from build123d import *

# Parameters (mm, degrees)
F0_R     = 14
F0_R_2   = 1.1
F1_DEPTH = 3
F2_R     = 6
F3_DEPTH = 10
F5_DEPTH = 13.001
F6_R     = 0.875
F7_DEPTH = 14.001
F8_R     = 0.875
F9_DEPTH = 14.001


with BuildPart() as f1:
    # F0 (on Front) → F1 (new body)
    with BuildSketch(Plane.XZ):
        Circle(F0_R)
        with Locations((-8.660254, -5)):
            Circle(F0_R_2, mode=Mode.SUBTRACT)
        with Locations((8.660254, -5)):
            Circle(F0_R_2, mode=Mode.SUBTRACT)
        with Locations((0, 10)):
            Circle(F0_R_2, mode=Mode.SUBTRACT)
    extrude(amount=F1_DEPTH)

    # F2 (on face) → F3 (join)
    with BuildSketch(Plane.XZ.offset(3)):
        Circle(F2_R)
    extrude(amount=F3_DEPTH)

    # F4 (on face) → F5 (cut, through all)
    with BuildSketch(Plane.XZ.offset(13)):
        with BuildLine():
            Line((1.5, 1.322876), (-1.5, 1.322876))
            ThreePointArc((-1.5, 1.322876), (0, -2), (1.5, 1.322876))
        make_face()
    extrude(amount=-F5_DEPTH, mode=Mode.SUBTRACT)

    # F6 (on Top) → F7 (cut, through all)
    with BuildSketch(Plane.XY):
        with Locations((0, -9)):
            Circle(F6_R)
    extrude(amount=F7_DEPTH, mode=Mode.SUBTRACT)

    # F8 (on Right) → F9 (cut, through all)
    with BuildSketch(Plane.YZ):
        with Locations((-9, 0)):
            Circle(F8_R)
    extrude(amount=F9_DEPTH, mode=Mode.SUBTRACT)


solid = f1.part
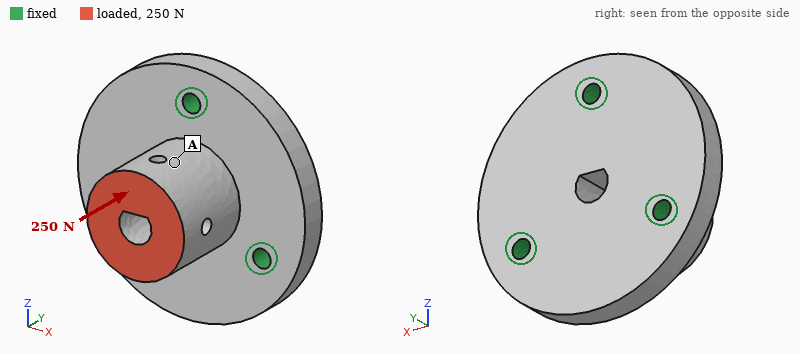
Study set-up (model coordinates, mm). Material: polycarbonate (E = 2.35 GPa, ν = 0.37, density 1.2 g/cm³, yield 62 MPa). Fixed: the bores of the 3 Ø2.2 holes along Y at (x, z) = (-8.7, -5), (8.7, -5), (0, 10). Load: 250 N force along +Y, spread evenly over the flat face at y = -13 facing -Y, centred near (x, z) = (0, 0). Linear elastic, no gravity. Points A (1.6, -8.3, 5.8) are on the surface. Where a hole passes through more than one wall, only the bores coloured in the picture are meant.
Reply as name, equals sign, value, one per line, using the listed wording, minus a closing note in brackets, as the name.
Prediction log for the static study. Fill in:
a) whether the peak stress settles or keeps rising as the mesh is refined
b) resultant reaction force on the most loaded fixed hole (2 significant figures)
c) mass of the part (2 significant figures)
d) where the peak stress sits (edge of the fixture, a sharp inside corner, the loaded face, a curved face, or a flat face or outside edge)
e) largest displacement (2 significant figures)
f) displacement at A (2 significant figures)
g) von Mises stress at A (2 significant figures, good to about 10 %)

whether the peak stress settles or keeps rising as the mesh is refined = keeps rising
resultant reaction force on the most loaded fixed hole = 86 N
mass of the part = 3.3 g
where the peak stress sits = edge of the fixture
largest displacement = 54 µm
displacement at A = 48 µm
von Mises stress at A = 3.4 MPa
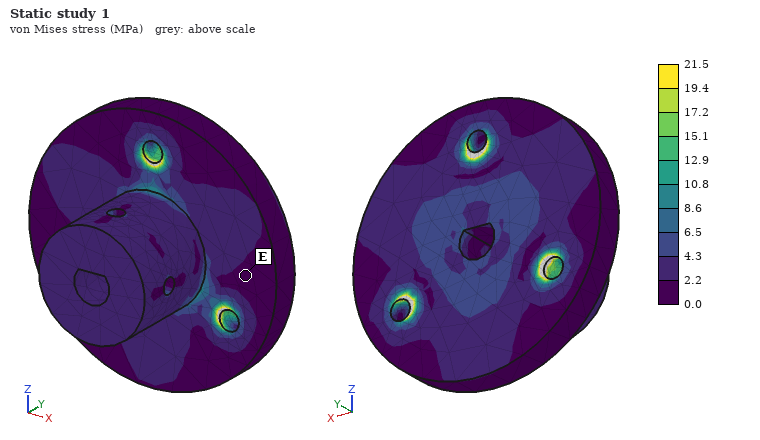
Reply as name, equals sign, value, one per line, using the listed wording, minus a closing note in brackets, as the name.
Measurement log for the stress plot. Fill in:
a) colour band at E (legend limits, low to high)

colour band at E = 0.0 to 2.2 MPa
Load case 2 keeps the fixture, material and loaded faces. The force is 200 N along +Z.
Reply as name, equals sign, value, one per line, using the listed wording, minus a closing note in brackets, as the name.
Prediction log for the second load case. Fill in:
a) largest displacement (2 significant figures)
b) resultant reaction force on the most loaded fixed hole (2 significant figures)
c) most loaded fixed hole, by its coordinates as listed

largest displacement = 0.21 mm
resultant reaction force on the most loaded fixed hole = 180 N
most loaded fixed hole, by its coordinates as listed = (0, 10)
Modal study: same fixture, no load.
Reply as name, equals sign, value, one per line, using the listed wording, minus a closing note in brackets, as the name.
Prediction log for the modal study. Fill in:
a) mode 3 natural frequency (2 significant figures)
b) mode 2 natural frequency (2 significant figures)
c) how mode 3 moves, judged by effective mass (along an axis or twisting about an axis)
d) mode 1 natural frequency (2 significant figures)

mode 3 natural frequency = 7800 Hz
mode 2 natural frequency = 6400 Hz
how mode 3 moves, judged by effective mass = along Y
mode 1 natural frequency = 6400 Hz
